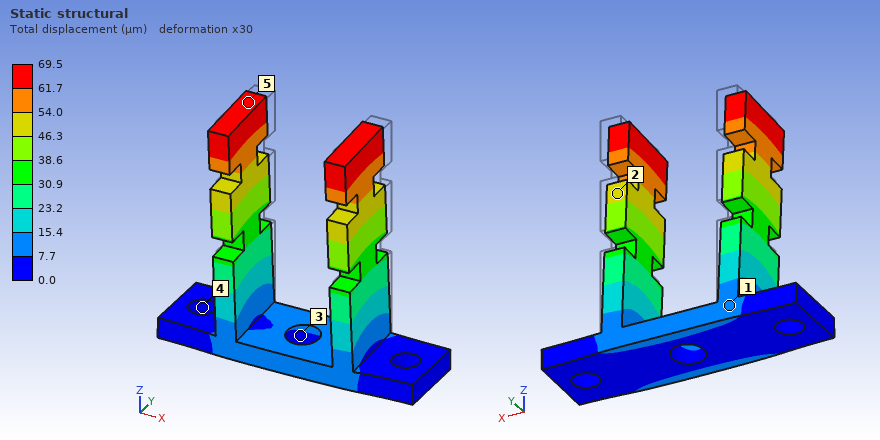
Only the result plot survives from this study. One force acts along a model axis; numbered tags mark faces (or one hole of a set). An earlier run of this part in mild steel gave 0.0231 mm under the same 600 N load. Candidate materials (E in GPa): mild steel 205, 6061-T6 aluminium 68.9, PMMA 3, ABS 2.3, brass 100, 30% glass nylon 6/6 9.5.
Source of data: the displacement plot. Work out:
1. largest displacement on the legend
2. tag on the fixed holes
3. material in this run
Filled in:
69.5 µm
4
6061-T6 aluminium
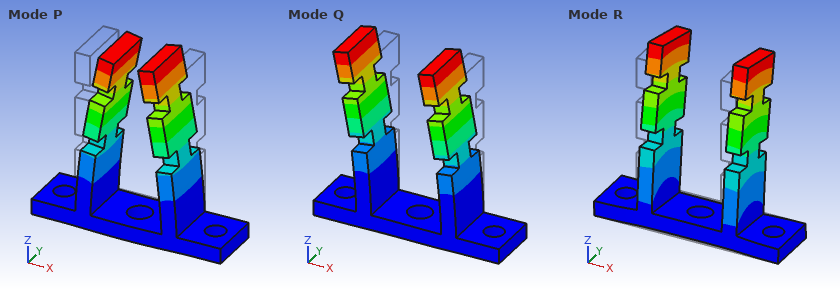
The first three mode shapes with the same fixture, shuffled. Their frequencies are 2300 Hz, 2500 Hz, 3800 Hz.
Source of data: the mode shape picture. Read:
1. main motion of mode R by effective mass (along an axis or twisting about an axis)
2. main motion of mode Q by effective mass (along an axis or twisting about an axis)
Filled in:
along Y
along X
